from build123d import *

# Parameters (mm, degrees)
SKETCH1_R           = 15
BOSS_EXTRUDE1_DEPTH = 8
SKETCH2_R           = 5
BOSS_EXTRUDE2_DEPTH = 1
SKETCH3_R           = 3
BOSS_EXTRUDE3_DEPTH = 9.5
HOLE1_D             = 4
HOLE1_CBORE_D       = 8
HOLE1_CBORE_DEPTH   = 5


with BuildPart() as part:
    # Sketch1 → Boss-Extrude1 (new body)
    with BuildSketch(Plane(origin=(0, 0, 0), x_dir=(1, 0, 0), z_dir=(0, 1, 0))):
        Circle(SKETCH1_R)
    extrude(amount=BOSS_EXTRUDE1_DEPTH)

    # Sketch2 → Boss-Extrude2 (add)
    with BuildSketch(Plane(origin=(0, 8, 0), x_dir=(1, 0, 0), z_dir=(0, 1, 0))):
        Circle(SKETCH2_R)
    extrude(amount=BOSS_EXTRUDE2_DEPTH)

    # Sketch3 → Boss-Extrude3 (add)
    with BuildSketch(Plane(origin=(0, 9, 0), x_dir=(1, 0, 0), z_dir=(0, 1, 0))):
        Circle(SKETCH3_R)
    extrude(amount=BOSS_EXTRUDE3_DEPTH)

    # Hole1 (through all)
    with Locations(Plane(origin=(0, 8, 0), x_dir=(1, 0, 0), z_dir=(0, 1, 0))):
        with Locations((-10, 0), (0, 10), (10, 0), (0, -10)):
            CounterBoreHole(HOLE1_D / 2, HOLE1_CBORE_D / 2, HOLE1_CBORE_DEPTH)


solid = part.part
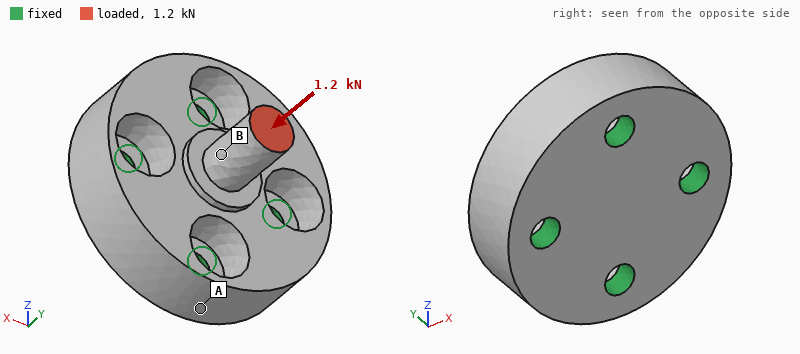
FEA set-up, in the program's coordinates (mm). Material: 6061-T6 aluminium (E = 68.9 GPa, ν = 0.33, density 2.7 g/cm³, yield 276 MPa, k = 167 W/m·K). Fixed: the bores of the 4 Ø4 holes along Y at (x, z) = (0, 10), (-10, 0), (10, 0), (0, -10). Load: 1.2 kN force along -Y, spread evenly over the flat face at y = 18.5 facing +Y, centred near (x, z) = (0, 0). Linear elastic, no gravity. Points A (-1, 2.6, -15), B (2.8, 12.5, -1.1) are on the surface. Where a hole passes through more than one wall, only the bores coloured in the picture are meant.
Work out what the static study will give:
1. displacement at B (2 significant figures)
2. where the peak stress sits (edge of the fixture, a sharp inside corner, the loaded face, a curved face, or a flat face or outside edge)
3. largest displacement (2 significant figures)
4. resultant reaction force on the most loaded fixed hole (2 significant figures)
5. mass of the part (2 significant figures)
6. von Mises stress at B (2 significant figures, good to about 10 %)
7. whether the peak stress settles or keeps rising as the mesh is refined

5.6 µm
edge of the fixture
9.3 µm
330 N
13 g
43 MPa
keeps rising
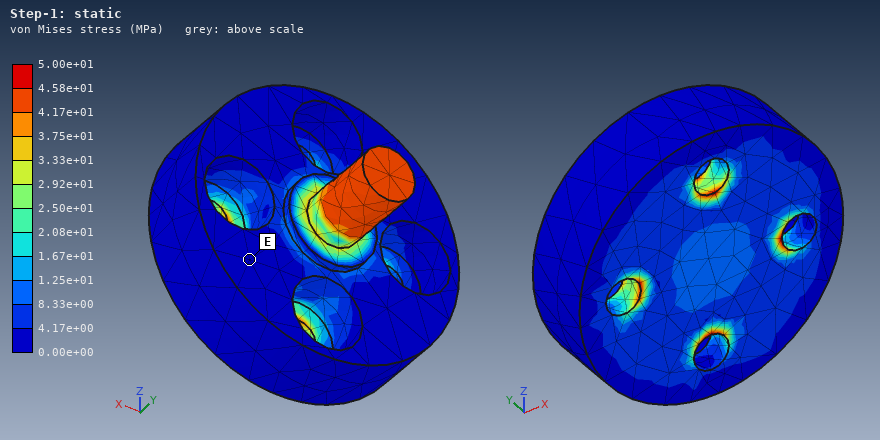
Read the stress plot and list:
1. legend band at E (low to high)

0.00e+00 to 4.17e+00 MPa
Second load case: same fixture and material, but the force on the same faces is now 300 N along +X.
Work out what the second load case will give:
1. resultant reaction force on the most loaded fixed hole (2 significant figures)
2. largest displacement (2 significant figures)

260 N
38 µm
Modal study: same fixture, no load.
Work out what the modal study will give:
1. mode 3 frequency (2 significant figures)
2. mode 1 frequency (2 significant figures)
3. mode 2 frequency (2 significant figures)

43 kHz
29 kHz
29 kHz
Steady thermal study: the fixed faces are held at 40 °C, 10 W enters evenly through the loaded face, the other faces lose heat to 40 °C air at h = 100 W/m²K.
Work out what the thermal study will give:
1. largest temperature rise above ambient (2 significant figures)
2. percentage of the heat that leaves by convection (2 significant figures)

25 K
4.9 %
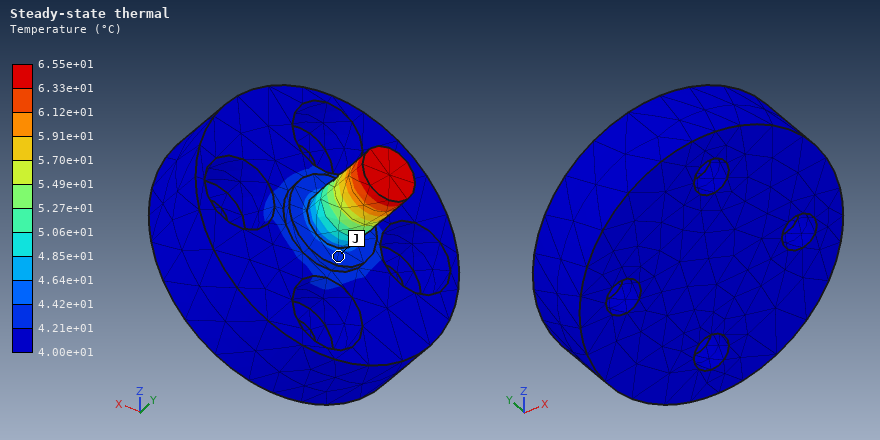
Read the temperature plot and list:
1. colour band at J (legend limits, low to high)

4.21e+01 to 4.42e+01 °C
